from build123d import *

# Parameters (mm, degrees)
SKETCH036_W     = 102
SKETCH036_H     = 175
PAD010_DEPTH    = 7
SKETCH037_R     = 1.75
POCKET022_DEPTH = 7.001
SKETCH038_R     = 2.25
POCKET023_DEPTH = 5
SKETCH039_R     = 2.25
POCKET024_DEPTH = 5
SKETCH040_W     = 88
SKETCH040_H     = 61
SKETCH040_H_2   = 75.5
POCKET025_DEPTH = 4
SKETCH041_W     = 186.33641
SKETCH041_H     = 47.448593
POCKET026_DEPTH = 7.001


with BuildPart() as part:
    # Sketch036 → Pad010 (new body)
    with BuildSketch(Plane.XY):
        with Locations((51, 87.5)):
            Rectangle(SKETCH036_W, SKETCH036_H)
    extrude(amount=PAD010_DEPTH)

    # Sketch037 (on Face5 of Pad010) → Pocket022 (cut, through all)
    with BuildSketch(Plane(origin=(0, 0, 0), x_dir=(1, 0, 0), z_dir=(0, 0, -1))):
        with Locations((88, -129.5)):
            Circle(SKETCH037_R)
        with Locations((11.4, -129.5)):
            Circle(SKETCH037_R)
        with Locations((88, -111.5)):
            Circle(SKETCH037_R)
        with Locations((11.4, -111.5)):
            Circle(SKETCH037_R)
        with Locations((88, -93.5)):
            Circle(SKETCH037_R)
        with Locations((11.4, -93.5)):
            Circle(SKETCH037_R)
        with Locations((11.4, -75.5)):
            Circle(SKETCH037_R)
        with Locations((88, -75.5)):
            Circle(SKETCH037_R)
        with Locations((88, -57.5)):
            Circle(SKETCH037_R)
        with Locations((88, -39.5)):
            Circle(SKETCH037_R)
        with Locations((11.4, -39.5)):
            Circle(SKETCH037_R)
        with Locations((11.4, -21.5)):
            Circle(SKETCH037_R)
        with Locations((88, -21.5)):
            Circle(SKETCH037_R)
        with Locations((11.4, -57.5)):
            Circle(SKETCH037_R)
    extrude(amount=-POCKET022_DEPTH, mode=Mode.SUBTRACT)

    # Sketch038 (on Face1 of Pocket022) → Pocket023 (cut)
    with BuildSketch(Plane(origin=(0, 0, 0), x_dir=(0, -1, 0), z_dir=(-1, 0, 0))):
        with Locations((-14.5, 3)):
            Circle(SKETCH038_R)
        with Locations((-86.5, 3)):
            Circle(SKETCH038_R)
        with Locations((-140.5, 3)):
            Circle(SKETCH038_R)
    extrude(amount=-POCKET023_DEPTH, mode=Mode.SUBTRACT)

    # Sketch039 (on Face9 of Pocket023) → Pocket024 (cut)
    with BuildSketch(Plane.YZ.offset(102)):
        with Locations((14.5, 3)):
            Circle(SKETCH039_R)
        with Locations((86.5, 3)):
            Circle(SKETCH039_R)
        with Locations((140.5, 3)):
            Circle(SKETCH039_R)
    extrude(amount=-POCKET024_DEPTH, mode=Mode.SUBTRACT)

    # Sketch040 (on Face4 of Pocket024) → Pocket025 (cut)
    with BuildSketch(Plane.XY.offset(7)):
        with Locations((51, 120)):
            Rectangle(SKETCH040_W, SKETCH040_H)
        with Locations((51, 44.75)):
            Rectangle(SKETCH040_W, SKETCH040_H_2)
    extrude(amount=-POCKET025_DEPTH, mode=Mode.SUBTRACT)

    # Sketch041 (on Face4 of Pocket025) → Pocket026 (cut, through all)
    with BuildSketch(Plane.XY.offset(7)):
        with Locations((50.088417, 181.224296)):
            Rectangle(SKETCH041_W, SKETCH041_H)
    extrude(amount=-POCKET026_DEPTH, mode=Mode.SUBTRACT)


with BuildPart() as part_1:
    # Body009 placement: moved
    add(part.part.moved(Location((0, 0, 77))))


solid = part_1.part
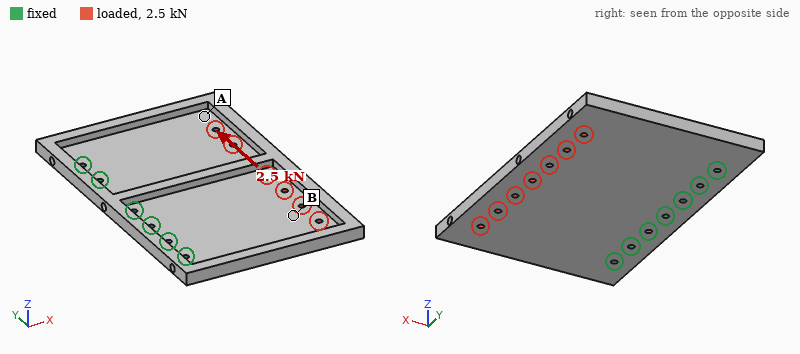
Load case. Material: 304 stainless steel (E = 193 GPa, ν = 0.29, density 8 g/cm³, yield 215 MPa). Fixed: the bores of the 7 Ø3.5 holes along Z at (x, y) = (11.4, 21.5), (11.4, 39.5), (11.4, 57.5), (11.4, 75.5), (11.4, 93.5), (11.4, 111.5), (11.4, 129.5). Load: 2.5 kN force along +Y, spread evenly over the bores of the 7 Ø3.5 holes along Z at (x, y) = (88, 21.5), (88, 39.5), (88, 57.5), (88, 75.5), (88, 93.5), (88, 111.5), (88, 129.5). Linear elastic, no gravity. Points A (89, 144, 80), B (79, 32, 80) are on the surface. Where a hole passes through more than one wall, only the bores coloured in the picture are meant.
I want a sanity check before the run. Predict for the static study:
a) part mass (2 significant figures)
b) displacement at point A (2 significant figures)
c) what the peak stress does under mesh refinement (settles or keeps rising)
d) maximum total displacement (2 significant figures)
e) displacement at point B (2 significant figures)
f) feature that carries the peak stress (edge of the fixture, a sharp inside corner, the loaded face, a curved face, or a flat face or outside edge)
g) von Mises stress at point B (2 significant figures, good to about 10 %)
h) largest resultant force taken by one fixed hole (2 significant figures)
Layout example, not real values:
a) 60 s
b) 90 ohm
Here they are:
a) 510 g
b) 12 µm
c) keeps rising
d) 14 µm
e) 10 µm
f) edge of the fixture
g) 10 MPa
h) 1.4 kN
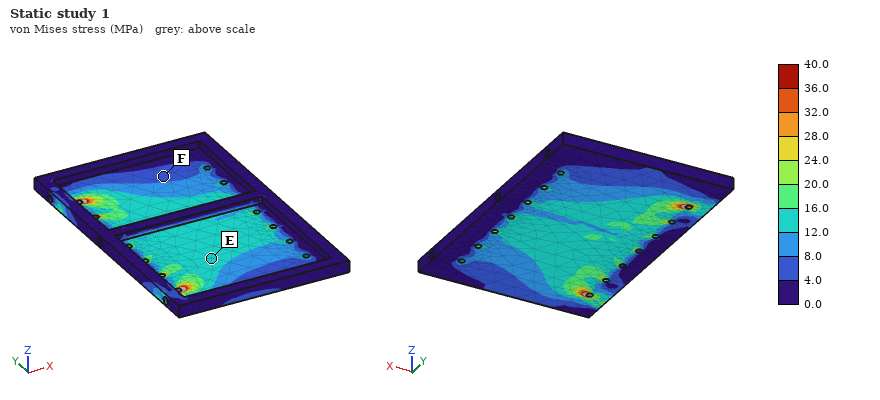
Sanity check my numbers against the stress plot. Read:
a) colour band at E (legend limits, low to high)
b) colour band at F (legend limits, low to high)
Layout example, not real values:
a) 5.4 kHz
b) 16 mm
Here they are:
a) 12.0 to 16.0 MPa
b) 4.0 to 8.0 MPa
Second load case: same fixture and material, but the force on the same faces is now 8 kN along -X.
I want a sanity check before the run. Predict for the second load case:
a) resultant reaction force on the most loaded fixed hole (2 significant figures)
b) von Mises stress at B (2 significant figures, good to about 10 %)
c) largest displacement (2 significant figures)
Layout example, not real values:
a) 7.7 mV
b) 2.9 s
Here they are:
a) 1.5 kN
b) 16 MPa
c) 40 µm
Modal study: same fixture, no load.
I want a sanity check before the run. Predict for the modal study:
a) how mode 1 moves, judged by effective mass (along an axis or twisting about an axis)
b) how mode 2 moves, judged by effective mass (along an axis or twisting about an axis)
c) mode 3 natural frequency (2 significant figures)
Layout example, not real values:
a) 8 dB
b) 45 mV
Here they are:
a) along Z
b) twisting about X
c) 1300 Hz
